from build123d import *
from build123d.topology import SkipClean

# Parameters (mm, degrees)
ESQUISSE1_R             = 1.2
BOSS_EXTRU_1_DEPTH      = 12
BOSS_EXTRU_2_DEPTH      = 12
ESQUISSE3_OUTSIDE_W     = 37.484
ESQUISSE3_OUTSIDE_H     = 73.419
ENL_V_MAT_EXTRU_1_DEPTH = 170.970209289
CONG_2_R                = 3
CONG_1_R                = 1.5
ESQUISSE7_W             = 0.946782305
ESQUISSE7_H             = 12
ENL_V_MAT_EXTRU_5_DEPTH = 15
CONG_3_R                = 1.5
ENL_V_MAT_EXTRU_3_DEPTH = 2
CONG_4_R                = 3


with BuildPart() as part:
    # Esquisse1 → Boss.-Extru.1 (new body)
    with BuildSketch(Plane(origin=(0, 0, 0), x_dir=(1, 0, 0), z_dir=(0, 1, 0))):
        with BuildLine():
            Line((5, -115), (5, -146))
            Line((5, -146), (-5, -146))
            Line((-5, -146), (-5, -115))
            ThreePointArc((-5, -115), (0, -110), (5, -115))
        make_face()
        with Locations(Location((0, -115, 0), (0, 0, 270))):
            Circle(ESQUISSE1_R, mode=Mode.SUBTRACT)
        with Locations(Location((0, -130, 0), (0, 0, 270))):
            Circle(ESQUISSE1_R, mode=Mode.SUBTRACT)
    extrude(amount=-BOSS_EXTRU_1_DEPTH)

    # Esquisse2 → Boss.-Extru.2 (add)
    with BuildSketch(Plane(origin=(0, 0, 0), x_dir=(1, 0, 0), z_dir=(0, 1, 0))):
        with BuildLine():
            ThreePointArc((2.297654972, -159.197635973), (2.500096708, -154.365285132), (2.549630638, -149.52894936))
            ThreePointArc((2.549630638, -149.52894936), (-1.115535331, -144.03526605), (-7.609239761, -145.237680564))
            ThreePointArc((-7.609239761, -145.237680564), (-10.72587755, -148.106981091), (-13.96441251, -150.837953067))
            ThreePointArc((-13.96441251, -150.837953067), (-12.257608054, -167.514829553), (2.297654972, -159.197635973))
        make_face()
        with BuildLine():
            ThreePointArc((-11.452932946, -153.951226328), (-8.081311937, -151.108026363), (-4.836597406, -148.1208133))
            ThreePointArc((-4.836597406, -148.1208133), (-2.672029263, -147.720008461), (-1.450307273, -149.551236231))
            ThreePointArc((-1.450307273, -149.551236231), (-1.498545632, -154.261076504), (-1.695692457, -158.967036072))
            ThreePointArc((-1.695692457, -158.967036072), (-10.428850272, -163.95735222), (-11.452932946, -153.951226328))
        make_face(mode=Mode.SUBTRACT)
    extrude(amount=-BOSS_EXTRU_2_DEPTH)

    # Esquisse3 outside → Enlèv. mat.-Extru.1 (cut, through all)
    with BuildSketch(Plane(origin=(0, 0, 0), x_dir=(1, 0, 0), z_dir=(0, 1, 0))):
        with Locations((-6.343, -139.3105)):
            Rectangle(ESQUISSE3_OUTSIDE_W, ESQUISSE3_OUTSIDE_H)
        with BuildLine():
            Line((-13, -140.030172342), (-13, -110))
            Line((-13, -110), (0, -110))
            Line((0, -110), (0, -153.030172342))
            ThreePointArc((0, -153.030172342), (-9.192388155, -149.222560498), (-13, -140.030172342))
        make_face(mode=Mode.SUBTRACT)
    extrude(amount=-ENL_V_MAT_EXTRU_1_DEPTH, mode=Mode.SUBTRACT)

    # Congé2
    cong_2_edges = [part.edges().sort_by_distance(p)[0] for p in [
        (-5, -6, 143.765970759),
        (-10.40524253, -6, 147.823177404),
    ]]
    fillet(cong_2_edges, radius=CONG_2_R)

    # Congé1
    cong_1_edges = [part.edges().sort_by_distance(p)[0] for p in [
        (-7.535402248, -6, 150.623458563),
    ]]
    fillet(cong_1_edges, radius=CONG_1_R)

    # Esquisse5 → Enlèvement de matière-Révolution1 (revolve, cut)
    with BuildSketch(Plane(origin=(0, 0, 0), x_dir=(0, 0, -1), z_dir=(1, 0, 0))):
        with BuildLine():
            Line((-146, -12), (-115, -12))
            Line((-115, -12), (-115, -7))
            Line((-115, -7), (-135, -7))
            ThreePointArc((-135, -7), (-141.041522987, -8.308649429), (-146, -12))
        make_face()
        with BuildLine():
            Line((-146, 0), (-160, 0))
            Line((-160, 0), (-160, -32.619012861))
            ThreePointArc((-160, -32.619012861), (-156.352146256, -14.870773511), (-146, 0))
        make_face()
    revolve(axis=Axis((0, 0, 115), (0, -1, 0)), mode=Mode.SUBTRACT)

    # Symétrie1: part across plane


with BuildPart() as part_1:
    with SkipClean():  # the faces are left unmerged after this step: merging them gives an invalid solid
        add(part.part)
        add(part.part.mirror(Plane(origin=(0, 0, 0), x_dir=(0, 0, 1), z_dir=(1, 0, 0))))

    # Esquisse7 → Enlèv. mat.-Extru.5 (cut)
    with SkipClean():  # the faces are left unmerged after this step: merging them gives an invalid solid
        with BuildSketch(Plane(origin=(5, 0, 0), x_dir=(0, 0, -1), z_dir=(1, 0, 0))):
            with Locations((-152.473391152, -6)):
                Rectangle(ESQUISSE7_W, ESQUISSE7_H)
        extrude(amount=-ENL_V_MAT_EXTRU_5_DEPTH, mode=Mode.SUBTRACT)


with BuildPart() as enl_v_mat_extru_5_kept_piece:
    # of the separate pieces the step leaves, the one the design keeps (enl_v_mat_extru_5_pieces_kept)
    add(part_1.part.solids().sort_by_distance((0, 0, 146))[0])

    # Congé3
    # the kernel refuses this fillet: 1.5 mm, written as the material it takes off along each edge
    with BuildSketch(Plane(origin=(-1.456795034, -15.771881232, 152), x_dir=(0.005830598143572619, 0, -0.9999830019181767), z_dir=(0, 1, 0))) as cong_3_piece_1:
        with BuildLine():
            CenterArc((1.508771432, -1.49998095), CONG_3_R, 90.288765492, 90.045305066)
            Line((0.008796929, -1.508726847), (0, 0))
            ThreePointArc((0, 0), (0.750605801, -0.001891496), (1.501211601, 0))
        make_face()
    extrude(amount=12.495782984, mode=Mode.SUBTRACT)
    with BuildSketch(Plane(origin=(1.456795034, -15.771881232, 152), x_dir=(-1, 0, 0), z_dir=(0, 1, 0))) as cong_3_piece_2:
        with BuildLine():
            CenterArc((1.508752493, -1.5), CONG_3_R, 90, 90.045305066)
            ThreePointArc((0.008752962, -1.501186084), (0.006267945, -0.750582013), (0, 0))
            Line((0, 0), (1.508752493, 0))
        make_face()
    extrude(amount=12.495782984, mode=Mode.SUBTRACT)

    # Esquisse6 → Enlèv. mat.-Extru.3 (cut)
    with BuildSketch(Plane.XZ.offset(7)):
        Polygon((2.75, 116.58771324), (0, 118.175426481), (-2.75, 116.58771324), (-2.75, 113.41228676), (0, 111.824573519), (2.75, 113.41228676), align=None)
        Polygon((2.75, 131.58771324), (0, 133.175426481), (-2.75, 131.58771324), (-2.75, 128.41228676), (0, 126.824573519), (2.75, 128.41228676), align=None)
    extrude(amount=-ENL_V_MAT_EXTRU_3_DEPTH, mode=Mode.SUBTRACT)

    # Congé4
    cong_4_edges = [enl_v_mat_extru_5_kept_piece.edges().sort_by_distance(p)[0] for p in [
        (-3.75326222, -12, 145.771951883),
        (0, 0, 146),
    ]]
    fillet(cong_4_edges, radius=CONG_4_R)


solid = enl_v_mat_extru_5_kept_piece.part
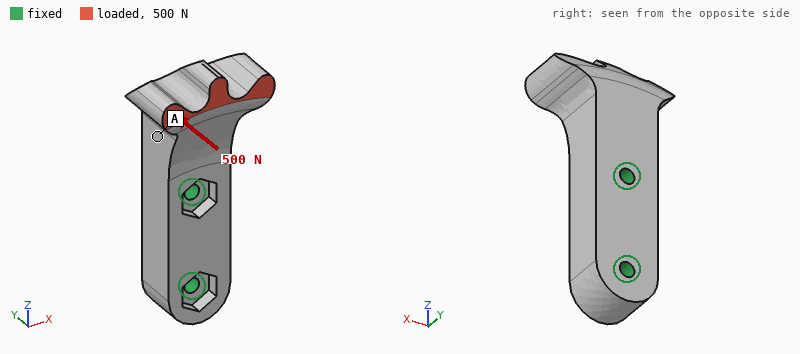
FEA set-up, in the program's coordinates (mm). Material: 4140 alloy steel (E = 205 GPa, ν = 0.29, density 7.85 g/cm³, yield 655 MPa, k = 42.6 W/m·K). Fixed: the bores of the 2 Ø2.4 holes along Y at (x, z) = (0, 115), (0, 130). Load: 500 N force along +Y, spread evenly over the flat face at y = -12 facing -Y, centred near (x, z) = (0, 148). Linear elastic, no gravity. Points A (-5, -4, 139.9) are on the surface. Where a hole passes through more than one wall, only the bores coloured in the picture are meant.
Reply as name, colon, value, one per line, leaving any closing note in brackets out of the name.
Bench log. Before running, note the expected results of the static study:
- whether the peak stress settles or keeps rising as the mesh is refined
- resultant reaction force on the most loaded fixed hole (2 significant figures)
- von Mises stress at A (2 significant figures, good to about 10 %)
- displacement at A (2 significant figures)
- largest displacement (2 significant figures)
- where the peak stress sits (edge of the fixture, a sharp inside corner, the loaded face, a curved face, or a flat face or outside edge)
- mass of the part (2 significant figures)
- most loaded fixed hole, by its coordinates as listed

whether the peak stress settles or keeps rising as the mesh is refined: keeps rising
resultant reaction force on the most loaded fixed hole: 790 N
von Mises stress at A: 28 MPa
displacement at A: 12 µm
largest displacement: 38 µm
where the peak stress sits: edge of the fixture
mass of the part: 25 g
most loaded fixed hole, by its coordinates as listed: (0, 130)
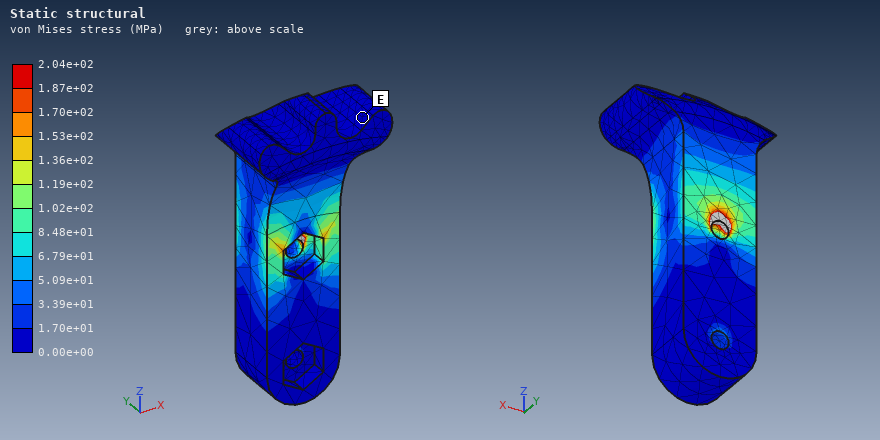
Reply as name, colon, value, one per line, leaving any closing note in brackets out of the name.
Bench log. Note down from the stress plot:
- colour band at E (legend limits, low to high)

colour band at E: 0.00e+00 to 1.70e+01 MPa
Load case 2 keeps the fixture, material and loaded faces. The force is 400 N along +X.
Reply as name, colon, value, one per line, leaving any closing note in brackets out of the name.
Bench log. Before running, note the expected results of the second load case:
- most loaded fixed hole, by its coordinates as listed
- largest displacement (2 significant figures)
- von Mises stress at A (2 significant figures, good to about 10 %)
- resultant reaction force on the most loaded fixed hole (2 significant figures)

most loaded fixed hole, by its coordinates as listed: (0, 130)
largest displacement: 27 µm
von Mises stress at A: 41 MPa
resultant reaction force on the most loaded fixed hole: 740 N
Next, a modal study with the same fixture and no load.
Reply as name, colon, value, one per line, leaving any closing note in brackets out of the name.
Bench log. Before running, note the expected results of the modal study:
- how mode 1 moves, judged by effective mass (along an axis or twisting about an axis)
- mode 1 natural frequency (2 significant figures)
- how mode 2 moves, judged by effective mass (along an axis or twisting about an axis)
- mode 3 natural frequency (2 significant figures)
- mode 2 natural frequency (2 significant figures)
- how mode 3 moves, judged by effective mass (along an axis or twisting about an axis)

how mode 1 moves, judged by effective mass: along Y
mode 1 natural frequency: 7800 Hz
how mode 2 moves, judged by effective mass: along X
mode 3 natural frequency: 17 kHz
mode 2 natural frequency: 9300 Hz
how mode 3 moves, judged by effective mass: twisting about Z
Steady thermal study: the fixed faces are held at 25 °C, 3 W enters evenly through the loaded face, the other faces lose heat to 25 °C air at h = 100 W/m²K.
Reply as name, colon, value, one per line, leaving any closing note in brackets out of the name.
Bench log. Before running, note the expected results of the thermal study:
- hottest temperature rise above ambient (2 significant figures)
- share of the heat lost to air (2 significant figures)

hottest temperature rise above ambient: 18 K
share of the heat lost to air: 33 %
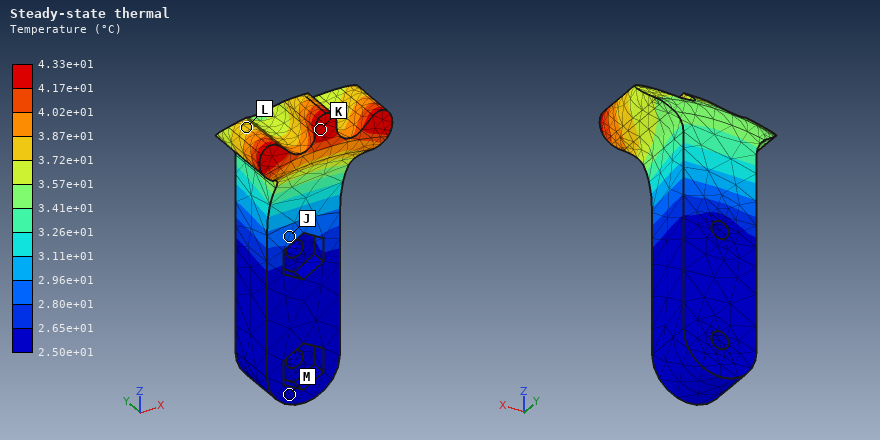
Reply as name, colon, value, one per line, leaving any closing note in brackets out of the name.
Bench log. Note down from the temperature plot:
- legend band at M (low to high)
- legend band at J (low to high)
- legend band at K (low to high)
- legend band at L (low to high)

legend band at M: 2.50e+01 to 2.65e+01 °C
legend band at J: 2.80e+01 to 2.96e+01 °C
legend band at K: 4.17e+01 to 4.33e+01 °C
legend band at L: 3.72e+01 to 3.87e+01 °C
